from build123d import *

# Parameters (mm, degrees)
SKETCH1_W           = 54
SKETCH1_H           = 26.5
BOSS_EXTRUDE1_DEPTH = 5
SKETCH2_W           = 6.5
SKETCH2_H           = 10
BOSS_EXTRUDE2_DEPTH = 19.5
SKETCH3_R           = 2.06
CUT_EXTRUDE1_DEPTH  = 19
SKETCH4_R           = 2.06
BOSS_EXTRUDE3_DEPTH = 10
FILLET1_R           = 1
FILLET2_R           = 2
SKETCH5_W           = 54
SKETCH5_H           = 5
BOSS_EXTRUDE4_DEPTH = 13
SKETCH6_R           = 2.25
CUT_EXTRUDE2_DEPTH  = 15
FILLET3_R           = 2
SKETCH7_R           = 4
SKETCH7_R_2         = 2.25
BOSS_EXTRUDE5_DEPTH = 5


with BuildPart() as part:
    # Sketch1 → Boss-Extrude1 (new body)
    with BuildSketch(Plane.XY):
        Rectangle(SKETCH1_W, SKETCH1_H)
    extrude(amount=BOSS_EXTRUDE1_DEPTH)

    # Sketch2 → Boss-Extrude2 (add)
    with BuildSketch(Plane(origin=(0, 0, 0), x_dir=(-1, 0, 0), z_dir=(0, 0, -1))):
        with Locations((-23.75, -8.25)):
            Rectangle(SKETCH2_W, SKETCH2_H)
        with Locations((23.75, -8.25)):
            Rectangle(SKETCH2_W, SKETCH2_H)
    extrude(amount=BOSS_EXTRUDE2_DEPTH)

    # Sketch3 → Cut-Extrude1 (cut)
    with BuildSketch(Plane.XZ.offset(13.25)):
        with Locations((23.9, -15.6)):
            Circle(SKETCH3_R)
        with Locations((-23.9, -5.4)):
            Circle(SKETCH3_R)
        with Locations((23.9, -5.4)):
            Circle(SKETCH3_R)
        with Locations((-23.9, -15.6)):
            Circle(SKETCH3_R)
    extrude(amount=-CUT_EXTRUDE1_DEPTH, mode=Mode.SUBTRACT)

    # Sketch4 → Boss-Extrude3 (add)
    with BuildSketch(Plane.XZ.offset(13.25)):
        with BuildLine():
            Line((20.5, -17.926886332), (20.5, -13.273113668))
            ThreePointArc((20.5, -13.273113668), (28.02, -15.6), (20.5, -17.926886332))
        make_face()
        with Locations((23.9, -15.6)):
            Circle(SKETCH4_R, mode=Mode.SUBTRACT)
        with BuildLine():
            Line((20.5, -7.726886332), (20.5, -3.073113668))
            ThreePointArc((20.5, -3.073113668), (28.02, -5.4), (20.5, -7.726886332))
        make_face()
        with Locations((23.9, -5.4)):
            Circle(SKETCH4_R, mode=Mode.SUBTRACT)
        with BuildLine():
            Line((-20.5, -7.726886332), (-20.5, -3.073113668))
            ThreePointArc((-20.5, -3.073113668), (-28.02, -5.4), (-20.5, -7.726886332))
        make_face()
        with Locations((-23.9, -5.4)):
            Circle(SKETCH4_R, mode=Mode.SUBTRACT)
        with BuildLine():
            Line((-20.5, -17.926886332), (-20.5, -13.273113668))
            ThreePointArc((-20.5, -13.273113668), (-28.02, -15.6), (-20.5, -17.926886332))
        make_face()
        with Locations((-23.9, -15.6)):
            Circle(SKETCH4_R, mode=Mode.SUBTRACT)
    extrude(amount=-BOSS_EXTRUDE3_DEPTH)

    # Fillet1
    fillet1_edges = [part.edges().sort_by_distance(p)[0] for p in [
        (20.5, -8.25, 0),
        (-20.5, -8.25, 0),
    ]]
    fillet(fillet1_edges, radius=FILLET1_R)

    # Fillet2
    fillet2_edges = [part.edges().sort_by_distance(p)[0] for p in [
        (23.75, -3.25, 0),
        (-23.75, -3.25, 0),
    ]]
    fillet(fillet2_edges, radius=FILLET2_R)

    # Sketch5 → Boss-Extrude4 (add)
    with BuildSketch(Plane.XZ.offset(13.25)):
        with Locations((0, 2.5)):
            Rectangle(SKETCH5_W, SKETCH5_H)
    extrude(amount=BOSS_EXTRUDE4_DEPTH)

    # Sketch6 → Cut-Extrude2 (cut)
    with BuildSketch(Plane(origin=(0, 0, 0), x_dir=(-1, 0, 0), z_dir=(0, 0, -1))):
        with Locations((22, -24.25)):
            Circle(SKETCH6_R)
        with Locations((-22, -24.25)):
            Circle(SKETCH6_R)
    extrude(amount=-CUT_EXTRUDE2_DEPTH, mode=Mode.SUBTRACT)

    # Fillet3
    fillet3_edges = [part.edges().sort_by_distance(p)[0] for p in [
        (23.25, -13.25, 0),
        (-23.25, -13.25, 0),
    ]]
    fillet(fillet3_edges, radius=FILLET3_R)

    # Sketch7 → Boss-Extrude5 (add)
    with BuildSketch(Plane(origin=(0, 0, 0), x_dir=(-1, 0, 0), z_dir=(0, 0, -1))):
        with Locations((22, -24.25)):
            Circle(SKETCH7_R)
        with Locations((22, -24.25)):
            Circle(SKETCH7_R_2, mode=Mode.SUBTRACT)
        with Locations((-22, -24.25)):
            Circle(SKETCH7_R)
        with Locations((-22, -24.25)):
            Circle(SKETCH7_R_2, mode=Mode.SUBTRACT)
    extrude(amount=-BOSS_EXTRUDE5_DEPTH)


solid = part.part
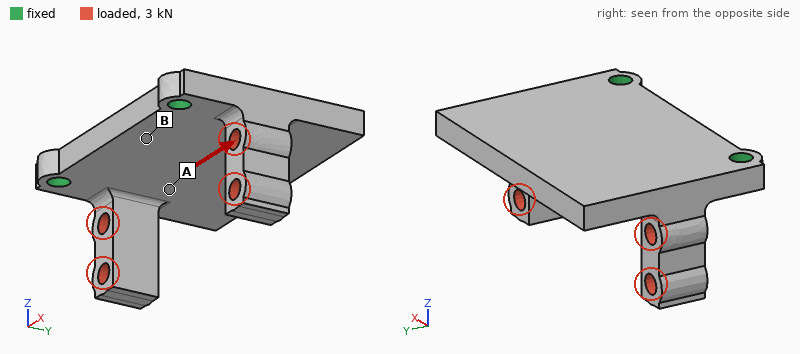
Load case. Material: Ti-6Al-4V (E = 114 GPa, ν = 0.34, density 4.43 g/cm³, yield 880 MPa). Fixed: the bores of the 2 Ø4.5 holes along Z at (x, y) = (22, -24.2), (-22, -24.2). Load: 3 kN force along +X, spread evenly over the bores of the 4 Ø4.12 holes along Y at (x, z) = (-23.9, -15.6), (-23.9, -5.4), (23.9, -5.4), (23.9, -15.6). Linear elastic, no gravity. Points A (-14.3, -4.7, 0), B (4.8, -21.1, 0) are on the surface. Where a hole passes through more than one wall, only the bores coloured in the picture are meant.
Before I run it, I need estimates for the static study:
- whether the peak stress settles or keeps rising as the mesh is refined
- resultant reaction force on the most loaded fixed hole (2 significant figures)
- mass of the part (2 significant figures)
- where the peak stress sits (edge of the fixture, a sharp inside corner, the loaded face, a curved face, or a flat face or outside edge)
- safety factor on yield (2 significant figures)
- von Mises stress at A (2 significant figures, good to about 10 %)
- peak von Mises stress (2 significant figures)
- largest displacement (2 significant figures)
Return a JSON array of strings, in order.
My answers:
["settles", "1.9 kN", "57 g", "a curved face", "1.7", "93 MPa", "510 MPa", "0.23 mm"]
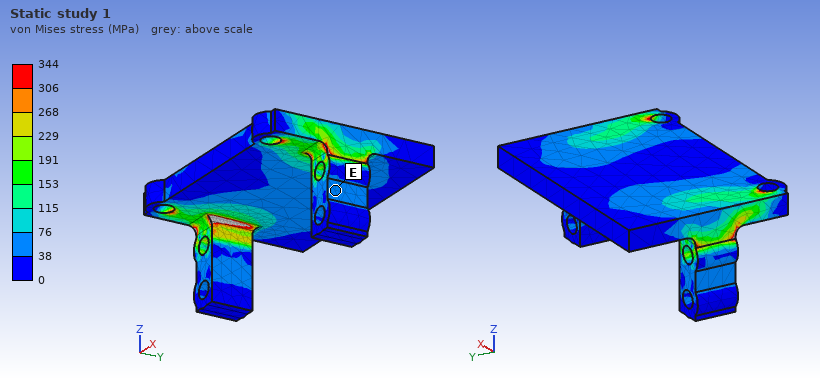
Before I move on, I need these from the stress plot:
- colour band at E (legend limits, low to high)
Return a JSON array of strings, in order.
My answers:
["38 to 76 MPa"]
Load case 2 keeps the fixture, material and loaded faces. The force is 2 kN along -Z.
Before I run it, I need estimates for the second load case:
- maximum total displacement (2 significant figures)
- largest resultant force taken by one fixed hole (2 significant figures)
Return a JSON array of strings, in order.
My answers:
["0.20 mm", "1.0 kN"]
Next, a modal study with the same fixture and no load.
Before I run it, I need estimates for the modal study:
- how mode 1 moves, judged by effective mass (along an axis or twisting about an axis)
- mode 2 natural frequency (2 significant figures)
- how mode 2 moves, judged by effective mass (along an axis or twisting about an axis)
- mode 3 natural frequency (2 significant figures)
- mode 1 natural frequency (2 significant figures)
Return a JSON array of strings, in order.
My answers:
["along Z", "4400 Hz", "twisting about Y", "6500 Hz", "2200 Hz"]
